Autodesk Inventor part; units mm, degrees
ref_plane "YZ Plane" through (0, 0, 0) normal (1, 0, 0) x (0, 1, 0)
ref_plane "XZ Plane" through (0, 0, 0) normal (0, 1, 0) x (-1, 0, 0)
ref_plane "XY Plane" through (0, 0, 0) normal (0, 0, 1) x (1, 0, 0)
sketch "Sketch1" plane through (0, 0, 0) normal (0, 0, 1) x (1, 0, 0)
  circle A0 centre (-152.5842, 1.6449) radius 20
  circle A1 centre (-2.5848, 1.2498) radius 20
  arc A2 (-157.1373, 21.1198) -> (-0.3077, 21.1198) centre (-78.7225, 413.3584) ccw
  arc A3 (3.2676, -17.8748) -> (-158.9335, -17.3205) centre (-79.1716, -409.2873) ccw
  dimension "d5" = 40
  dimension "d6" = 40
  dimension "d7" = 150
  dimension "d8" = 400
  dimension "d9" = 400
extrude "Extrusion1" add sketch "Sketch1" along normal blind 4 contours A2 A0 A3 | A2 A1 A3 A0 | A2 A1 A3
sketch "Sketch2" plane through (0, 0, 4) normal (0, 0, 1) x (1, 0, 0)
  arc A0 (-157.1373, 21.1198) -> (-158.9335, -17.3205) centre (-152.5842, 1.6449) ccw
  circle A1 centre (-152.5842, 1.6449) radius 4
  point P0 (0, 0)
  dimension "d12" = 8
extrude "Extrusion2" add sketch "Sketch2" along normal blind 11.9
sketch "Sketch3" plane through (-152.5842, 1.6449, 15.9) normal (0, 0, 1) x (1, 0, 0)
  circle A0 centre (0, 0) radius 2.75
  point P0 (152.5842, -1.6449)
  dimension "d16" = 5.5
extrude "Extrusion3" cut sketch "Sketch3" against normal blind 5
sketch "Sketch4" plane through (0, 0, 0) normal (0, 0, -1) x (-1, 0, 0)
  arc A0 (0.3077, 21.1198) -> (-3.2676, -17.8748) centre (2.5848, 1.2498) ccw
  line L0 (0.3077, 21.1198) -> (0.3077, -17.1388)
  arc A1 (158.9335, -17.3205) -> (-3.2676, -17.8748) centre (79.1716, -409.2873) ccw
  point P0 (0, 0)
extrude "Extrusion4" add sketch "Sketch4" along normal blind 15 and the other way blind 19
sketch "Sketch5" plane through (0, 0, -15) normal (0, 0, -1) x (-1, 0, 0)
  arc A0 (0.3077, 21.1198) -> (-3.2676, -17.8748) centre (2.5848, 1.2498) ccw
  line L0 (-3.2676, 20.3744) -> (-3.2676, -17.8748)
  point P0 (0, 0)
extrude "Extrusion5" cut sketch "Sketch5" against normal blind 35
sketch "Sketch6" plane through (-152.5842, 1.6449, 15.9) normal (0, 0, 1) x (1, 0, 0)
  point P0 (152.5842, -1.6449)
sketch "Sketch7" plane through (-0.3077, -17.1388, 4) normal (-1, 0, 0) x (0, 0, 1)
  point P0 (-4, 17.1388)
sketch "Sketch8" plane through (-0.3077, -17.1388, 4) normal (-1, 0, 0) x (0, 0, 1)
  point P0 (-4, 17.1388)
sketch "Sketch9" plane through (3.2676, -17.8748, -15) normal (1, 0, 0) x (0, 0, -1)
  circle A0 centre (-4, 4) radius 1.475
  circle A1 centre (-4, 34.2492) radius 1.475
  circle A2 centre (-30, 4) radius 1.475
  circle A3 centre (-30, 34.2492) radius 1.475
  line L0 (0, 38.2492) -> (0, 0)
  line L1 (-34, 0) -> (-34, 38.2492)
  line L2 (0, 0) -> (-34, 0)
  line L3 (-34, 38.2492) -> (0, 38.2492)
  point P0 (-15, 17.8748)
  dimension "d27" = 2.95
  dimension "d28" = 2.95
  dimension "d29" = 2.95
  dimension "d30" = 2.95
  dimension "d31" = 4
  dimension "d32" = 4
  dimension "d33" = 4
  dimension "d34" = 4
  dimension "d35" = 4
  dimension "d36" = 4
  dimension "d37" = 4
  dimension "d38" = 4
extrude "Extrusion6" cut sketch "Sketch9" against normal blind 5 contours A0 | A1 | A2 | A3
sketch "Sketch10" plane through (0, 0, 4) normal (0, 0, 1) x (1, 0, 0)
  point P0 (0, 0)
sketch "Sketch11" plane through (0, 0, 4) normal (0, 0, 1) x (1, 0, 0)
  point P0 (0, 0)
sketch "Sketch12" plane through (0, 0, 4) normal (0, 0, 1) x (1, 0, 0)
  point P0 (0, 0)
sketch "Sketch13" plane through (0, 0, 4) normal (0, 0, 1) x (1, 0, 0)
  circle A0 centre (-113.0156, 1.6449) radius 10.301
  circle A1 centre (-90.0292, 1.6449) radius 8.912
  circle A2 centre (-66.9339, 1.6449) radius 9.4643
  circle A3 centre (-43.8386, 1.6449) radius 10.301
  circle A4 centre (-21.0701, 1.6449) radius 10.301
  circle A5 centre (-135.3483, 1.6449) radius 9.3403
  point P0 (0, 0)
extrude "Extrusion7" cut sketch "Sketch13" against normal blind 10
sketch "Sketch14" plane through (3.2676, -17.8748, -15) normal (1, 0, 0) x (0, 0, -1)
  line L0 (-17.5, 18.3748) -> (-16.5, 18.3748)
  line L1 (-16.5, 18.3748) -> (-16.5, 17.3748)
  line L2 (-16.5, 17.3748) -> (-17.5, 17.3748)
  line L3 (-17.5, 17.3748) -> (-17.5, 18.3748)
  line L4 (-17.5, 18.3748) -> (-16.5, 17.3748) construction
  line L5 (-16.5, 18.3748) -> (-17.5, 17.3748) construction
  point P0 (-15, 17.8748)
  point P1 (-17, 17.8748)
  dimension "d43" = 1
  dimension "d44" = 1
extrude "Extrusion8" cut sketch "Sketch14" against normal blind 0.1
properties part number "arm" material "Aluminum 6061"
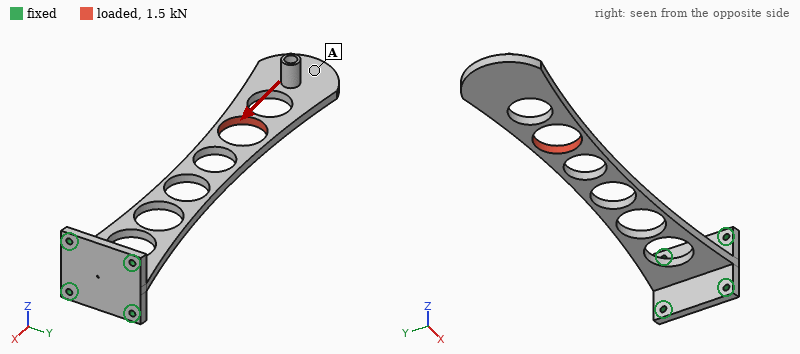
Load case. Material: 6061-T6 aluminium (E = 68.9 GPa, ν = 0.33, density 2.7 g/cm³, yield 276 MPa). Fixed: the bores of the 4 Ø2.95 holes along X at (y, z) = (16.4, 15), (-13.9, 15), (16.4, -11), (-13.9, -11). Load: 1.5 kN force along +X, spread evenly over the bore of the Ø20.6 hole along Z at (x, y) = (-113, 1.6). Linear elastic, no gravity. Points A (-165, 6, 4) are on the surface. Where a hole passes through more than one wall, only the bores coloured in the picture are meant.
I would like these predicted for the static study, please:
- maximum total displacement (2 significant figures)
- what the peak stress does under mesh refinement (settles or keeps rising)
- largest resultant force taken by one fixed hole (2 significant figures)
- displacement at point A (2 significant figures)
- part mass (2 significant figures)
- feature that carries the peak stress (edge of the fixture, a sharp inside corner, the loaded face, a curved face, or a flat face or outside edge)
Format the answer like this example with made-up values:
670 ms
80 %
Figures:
0.18 mm
keeps rising
390 N
0.16 mm
46 g
edge of the fixture
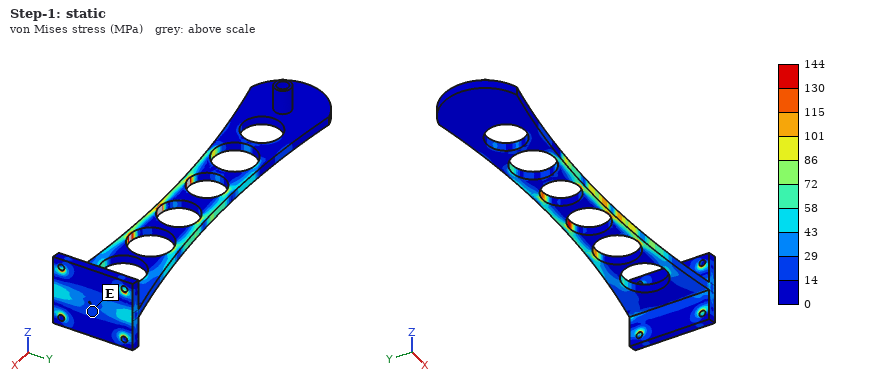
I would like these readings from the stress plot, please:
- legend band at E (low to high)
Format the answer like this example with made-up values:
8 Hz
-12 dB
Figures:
14 to 29 MPa
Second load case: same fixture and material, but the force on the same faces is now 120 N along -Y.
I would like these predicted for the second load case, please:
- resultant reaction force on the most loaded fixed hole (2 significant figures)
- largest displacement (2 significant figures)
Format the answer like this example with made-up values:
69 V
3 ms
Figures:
230 N
0.56 mm
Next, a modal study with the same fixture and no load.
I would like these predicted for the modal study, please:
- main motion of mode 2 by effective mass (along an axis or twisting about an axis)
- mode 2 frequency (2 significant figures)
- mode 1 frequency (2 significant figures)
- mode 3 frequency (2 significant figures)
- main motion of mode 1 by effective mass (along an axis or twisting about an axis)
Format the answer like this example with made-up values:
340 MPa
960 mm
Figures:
along Y
490 Hz
70 Hz
580 Hz
along Z
